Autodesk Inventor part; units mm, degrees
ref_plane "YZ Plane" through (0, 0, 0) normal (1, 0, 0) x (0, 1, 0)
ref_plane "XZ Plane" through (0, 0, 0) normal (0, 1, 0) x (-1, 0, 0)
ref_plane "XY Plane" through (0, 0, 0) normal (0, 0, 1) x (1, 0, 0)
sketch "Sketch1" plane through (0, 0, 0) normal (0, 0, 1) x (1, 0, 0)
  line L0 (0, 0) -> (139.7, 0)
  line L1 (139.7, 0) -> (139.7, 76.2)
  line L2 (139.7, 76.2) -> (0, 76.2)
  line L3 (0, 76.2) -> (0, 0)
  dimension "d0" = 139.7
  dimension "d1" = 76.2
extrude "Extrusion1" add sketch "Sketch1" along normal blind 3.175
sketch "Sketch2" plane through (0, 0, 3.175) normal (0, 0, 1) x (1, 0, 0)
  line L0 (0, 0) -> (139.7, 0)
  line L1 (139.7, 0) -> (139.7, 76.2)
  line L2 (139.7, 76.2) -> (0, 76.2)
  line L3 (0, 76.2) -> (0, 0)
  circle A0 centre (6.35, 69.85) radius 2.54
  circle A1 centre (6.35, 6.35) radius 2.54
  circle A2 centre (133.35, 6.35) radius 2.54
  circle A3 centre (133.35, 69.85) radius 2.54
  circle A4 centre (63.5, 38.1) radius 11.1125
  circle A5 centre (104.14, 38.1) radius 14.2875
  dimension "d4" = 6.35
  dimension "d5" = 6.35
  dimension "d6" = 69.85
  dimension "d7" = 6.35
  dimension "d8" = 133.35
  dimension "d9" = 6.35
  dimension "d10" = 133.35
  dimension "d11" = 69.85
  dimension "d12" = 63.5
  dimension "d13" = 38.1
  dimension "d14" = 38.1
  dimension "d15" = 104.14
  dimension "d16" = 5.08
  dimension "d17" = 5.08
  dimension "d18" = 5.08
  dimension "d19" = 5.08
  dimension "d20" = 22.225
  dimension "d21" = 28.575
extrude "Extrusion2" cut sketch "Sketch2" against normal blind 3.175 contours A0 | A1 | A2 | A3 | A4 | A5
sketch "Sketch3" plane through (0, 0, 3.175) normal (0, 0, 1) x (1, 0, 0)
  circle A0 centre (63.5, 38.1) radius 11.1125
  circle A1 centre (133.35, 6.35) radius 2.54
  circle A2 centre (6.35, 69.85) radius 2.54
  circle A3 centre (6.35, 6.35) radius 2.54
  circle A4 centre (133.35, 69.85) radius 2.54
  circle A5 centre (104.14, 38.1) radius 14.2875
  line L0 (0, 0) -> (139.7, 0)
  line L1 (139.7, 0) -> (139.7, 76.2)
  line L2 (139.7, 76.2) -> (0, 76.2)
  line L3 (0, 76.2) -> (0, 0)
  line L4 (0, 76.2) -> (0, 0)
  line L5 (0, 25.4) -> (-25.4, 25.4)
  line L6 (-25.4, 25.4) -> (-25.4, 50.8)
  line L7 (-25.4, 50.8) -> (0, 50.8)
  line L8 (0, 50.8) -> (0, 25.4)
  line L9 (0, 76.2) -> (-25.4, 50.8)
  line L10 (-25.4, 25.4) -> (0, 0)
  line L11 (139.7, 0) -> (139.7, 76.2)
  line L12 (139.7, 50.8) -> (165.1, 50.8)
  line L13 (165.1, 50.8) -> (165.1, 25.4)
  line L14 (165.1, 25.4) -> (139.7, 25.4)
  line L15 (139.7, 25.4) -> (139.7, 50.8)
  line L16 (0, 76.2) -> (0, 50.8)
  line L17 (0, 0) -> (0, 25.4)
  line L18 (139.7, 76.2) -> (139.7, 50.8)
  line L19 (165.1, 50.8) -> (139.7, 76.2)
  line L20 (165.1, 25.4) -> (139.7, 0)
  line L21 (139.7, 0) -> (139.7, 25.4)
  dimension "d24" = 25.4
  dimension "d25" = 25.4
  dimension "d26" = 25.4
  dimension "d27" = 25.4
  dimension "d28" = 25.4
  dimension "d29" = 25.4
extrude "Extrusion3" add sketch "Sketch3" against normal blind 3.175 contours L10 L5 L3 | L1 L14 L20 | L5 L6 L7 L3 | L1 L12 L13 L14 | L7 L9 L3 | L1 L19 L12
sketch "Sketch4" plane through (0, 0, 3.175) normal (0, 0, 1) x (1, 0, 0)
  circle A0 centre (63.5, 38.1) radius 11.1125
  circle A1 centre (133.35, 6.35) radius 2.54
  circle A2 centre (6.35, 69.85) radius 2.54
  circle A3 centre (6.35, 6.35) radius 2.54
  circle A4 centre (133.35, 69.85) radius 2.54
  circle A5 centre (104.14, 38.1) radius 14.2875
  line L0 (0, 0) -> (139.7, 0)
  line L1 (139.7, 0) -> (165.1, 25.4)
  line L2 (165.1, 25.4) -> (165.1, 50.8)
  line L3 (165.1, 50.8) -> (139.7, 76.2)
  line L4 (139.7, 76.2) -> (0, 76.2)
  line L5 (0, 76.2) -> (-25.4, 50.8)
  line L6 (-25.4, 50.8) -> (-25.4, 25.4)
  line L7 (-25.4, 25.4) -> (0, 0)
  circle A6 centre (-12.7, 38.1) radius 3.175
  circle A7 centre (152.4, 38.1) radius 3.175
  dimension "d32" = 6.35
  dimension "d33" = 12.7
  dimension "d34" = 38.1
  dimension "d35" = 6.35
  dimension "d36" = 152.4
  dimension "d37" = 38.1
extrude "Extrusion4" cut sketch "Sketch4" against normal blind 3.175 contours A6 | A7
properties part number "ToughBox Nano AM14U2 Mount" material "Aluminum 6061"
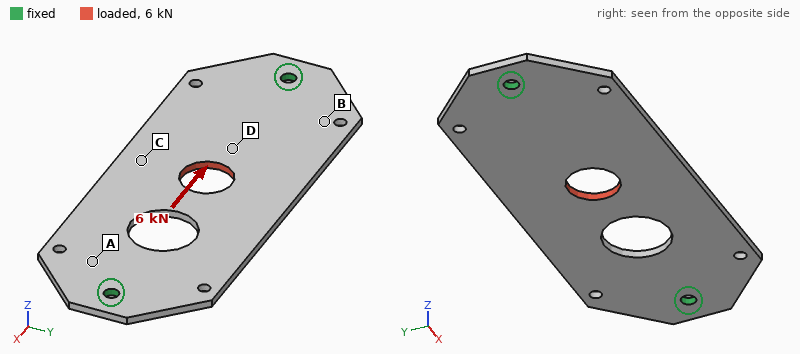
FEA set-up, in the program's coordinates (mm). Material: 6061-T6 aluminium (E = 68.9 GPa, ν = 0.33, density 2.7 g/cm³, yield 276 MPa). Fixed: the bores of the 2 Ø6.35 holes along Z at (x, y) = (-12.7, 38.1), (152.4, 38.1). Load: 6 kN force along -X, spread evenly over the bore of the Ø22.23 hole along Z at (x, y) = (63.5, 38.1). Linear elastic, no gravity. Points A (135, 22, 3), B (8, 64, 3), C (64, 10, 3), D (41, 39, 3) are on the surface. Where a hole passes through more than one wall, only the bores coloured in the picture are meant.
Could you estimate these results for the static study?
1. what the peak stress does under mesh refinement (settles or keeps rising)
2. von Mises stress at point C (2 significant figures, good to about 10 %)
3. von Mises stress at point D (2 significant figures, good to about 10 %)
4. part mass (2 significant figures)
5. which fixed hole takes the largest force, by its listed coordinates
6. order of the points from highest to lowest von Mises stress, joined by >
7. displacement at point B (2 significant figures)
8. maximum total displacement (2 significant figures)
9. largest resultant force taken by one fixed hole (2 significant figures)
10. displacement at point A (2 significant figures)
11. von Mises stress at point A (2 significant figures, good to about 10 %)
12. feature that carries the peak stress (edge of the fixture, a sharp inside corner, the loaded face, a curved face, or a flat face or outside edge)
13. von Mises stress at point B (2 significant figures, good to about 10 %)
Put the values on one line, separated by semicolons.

keeps rising; 4.9 MPa; 28 MPa; 100 g; (-12.7, 38.1); D > A > B > C; 17 µm; 40 µm; 3.6 kN; 10 µm; 19 MPa; edge of the fixture; 11 MPa
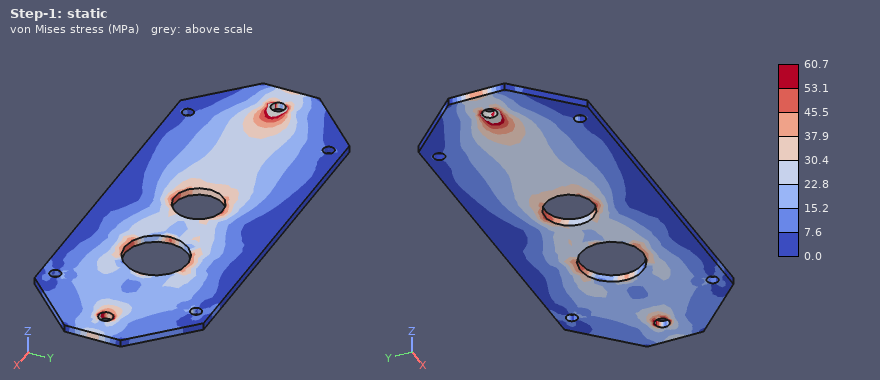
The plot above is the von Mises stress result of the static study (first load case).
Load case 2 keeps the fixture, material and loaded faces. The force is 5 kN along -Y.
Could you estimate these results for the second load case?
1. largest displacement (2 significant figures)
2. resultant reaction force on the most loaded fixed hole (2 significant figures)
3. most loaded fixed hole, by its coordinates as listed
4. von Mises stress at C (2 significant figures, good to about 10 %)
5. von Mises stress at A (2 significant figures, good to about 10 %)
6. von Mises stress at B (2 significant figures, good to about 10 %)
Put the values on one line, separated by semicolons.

0.11 mm; 2.7 kN; (-12.7, 38.1); 45 MPa; 22 MPa; 20 MPa
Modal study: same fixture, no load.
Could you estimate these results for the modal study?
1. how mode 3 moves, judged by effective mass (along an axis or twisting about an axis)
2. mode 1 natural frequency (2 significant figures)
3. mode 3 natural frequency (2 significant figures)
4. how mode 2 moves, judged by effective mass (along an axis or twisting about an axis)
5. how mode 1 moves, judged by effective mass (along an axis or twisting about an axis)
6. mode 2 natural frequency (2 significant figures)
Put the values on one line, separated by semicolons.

twisting about Y; 540 Hz; 1400 Hz; twisting about X; along Z; 680 Hz
